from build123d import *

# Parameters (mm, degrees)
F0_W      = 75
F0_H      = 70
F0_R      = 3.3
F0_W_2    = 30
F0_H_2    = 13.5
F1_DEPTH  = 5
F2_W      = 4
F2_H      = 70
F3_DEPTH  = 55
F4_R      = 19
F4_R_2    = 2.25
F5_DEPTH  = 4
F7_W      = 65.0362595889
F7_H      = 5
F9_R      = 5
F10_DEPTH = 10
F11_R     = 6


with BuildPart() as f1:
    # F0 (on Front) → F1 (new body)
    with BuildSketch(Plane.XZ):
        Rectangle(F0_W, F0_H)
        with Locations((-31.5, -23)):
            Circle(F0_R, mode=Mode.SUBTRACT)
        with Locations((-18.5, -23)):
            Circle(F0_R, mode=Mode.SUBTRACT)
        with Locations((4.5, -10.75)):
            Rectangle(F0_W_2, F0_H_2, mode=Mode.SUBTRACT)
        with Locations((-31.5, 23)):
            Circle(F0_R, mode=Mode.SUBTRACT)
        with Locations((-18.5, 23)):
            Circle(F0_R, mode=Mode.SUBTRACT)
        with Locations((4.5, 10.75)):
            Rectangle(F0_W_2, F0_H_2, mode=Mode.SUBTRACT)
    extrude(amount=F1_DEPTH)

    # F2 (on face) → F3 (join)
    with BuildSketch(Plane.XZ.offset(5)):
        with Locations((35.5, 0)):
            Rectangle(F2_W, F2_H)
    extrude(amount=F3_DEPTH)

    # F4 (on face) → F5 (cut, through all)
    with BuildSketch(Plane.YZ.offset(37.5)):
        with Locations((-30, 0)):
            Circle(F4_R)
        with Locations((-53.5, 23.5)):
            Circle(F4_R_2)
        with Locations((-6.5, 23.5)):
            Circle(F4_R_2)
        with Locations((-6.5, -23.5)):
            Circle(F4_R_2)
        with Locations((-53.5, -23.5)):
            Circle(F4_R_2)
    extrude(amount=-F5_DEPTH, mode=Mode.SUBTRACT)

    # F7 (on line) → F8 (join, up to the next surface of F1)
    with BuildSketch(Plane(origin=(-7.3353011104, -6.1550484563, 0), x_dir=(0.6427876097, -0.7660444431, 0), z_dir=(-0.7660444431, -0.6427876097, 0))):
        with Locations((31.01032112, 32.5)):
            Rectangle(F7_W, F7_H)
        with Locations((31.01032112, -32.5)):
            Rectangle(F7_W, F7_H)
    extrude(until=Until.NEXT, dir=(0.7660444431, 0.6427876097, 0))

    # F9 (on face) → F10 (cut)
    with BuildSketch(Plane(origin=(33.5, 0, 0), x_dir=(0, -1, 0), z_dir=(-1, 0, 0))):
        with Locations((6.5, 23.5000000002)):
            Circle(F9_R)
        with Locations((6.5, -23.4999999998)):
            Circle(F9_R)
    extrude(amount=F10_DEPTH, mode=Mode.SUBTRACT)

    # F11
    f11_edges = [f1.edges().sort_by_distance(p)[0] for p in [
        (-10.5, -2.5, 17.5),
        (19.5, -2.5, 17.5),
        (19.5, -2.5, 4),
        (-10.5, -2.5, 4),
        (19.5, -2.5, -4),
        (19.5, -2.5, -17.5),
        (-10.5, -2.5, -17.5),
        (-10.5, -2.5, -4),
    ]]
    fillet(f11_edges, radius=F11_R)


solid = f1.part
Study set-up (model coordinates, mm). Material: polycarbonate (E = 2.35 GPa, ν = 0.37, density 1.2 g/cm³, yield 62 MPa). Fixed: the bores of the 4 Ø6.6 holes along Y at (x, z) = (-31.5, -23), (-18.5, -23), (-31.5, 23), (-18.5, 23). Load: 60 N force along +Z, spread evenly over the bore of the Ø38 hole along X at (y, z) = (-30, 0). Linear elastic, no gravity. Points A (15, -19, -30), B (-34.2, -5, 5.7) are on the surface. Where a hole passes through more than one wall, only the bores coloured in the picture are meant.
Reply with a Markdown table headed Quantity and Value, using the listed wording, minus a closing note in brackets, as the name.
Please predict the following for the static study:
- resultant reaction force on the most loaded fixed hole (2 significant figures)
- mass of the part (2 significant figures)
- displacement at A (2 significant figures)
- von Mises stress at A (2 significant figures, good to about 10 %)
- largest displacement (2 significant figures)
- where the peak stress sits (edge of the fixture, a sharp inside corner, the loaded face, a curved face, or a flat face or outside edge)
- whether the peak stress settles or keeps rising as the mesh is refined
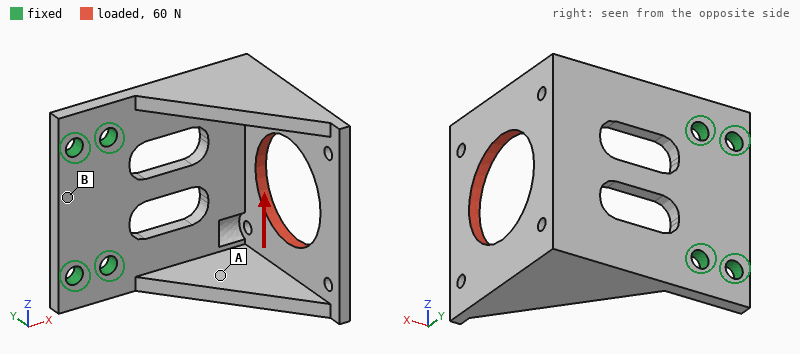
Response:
| Quantity | Value |
|---|---|
| resultant reaction force on the most loaded fixed hole | 61 N |
| mass of the part | 51 g |
| displacement at A | 0.38 mm |
| von Mises stress at A | 1.3 MPa |
| largest displacement | 1.1 mm |
| where the peak stress sits | edge of the fixture |
| whether the peak stress settles or keeps rising as the mesh is refined | keeps rising |
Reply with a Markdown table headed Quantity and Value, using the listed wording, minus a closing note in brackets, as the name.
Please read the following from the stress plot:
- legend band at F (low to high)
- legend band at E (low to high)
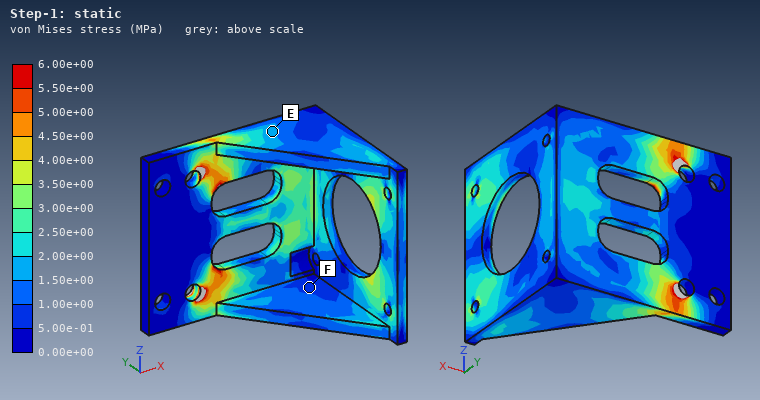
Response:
| Quantity | Value |
|---|---|
| legend band at F | 5.00e-01 to 1.00e+00 MPa |
| legend band at E | 1.50e+00 to 2.00e+00 MPa |
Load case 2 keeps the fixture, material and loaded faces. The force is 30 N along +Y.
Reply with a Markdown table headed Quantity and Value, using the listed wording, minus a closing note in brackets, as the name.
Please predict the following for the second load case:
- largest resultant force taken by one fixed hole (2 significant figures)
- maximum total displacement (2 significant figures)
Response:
| Quantity | Value |
|---|---|
| largest resultant force taken by one fixed hole | 31 N |
| maximum total displacement | 1.4 mm |
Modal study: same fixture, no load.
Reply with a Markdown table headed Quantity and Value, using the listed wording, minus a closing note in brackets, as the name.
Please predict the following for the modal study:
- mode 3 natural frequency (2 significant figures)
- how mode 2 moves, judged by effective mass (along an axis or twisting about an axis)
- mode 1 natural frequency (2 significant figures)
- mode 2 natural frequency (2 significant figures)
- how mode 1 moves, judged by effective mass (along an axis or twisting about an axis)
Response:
| Quantity | Value |
|---|---|
| mode 3 natural frequency | 910 Hz |
| how mode 2 moves, judged by effective mass | along Z |
| mode 1 natural frequency | 160 Hz |
| mode 2 natural frequency | 250 Hz |
| how mode 1 moves, judged by effective mass | along Y |
